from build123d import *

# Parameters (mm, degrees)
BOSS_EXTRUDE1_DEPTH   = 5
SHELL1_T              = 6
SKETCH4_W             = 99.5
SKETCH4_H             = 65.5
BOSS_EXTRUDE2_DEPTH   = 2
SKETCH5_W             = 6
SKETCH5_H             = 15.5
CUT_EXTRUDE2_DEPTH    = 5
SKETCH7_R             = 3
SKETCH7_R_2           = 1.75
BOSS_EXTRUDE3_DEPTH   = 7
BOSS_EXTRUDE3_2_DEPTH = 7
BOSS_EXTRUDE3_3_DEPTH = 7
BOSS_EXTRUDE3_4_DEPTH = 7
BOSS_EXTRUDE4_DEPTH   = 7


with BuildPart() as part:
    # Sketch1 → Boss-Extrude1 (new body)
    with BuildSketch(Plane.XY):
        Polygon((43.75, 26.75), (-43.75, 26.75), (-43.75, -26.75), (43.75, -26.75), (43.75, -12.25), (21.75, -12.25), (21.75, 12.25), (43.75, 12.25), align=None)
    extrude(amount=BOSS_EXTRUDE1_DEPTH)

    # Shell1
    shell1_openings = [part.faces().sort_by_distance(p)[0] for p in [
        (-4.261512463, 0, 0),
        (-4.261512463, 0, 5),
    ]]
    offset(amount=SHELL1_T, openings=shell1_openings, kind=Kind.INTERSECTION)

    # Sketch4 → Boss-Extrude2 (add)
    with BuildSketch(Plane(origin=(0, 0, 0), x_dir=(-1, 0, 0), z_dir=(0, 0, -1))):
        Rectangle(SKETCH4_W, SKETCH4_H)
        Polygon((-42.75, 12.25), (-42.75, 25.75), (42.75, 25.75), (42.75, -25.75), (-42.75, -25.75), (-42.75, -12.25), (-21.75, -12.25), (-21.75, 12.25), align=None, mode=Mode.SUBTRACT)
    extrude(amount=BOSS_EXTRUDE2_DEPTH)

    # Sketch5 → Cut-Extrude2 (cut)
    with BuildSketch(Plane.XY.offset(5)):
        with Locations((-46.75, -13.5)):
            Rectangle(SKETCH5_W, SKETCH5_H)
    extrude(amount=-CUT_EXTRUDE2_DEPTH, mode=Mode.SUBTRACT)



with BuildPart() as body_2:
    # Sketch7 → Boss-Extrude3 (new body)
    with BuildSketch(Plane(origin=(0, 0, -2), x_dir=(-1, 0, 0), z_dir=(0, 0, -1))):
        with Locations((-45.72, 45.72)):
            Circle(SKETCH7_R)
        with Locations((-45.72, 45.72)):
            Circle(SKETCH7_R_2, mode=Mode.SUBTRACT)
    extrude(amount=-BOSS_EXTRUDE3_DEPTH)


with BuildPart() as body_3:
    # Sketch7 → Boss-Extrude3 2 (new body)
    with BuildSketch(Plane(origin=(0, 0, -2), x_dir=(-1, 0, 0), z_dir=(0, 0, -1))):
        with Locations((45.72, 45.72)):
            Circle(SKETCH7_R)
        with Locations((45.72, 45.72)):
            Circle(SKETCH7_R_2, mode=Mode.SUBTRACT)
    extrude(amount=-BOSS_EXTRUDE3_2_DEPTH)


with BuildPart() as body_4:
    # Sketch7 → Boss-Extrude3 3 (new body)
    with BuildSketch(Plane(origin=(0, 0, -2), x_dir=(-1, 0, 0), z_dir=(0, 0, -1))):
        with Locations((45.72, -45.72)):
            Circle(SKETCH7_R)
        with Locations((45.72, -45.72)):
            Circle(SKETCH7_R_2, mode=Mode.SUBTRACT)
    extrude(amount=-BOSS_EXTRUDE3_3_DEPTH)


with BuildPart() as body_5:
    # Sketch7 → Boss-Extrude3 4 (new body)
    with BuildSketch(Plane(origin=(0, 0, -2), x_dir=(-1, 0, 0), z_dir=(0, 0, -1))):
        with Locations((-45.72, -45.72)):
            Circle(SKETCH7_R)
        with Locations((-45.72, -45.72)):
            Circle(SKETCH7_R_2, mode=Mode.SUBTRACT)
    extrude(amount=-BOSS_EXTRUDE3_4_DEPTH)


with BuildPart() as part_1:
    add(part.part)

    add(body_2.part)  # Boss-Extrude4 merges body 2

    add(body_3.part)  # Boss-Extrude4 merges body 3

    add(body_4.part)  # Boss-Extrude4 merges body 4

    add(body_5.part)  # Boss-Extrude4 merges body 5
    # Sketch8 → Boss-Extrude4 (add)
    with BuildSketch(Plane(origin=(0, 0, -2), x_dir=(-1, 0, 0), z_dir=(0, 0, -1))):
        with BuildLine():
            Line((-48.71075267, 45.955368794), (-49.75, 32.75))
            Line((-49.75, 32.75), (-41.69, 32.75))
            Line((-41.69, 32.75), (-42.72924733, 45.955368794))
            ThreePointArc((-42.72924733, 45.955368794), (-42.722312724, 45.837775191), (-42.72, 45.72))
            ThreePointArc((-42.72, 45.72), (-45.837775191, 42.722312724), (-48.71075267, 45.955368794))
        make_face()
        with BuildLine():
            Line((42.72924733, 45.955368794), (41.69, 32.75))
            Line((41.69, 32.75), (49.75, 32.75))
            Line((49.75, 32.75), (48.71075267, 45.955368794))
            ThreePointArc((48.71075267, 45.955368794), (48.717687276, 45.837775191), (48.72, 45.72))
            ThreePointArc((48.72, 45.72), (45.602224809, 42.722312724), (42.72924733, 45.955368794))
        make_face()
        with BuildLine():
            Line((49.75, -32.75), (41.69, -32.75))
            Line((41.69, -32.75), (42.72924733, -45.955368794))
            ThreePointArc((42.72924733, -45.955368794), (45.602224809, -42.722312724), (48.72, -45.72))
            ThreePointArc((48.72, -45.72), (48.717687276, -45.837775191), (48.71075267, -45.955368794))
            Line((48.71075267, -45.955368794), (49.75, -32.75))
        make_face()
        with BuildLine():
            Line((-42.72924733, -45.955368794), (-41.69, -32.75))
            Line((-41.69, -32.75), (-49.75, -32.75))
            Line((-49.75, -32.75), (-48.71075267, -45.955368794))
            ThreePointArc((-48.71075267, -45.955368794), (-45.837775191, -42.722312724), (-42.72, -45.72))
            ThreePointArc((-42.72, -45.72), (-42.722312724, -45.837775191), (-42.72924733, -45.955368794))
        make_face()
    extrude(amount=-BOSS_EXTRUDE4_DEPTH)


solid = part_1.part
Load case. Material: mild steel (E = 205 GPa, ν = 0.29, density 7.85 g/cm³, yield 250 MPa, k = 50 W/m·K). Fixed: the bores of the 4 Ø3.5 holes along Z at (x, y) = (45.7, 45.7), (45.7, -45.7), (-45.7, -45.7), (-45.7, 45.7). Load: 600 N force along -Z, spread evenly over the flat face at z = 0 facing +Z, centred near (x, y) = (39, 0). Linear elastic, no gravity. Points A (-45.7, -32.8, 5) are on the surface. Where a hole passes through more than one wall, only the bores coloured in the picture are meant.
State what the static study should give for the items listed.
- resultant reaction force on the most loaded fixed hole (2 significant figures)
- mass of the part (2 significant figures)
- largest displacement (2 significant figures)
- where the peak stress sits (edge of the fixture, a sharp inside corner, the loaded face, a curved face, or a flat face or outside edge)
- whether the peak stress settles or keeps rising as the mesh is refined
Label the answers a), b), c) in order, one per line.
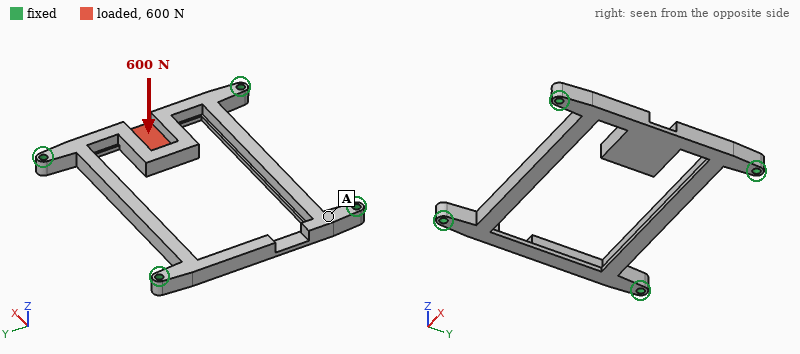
a) 780 N
b) 140 g
c) 0.14 mm
d) edge of the fixture
e) keeps rising
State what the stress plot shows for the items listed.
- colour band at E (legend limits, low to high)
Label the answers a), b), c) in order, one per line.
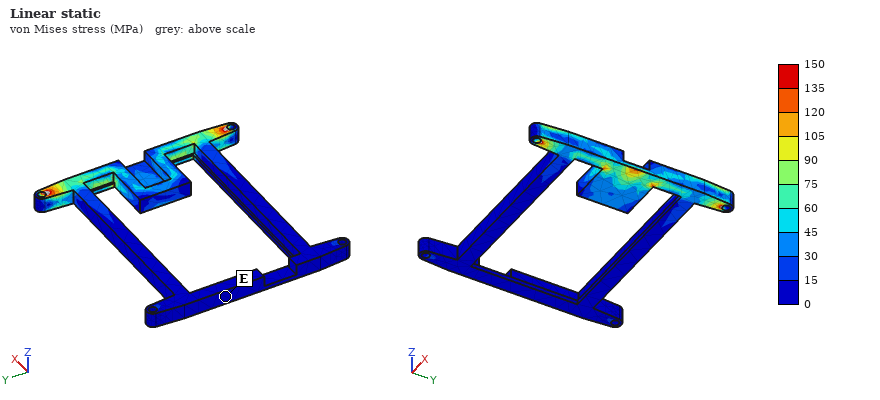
a) 0 to 15 MPa
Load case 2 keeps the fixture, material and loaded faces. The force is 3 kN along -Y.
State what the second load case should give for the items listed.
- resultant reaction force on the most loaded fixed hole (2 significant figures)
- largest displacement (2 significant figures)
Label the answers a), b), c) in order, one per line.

a) 1.5 kN
b) 50 µm
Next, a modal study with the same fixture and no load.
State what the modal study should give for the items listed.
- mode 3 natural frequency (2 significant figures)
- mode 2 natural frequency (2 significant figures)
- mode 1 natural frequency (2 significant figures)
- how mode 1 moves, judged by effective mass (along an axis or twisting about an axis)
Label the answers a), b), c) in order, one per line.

a) 3100 Hz
b) 3000 Hz
c) 2000 Hz
d) along Z
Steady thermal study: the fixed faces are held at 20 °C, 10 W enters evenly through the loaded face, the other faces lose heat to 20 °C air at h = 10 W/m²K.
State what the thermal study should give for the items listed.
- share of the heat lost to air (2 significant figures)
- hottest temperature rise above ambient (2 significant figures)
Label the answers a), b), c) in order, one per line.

a) 22 %
b) 75 K
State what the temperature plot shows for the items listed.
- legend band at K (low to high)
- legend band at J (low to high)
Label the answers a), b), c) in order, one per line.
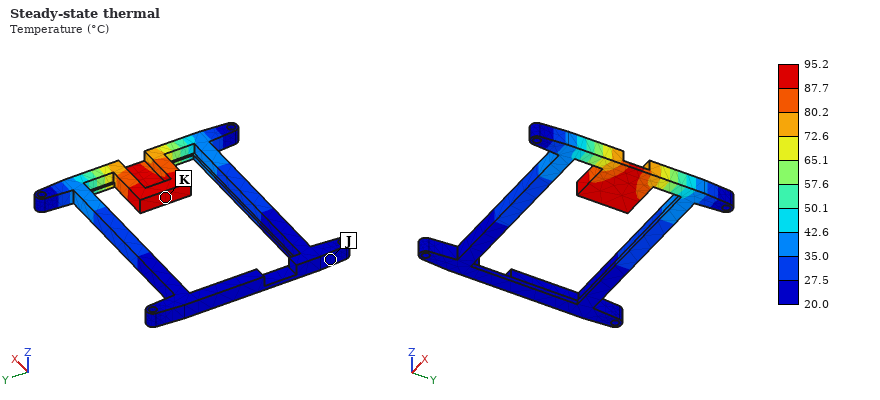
a) 87.7 to 95.2 °C
b) 20.0 to 27.5 °C
